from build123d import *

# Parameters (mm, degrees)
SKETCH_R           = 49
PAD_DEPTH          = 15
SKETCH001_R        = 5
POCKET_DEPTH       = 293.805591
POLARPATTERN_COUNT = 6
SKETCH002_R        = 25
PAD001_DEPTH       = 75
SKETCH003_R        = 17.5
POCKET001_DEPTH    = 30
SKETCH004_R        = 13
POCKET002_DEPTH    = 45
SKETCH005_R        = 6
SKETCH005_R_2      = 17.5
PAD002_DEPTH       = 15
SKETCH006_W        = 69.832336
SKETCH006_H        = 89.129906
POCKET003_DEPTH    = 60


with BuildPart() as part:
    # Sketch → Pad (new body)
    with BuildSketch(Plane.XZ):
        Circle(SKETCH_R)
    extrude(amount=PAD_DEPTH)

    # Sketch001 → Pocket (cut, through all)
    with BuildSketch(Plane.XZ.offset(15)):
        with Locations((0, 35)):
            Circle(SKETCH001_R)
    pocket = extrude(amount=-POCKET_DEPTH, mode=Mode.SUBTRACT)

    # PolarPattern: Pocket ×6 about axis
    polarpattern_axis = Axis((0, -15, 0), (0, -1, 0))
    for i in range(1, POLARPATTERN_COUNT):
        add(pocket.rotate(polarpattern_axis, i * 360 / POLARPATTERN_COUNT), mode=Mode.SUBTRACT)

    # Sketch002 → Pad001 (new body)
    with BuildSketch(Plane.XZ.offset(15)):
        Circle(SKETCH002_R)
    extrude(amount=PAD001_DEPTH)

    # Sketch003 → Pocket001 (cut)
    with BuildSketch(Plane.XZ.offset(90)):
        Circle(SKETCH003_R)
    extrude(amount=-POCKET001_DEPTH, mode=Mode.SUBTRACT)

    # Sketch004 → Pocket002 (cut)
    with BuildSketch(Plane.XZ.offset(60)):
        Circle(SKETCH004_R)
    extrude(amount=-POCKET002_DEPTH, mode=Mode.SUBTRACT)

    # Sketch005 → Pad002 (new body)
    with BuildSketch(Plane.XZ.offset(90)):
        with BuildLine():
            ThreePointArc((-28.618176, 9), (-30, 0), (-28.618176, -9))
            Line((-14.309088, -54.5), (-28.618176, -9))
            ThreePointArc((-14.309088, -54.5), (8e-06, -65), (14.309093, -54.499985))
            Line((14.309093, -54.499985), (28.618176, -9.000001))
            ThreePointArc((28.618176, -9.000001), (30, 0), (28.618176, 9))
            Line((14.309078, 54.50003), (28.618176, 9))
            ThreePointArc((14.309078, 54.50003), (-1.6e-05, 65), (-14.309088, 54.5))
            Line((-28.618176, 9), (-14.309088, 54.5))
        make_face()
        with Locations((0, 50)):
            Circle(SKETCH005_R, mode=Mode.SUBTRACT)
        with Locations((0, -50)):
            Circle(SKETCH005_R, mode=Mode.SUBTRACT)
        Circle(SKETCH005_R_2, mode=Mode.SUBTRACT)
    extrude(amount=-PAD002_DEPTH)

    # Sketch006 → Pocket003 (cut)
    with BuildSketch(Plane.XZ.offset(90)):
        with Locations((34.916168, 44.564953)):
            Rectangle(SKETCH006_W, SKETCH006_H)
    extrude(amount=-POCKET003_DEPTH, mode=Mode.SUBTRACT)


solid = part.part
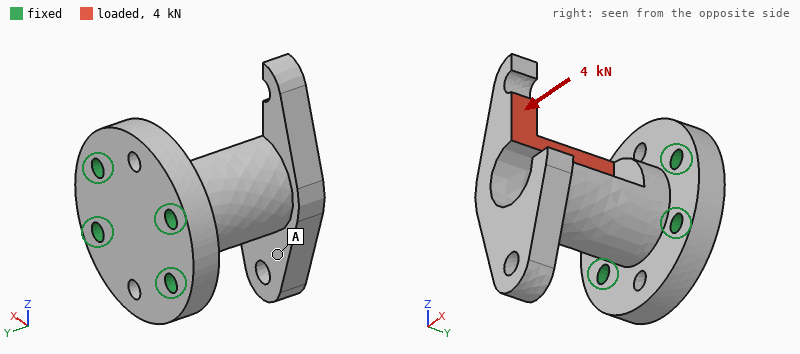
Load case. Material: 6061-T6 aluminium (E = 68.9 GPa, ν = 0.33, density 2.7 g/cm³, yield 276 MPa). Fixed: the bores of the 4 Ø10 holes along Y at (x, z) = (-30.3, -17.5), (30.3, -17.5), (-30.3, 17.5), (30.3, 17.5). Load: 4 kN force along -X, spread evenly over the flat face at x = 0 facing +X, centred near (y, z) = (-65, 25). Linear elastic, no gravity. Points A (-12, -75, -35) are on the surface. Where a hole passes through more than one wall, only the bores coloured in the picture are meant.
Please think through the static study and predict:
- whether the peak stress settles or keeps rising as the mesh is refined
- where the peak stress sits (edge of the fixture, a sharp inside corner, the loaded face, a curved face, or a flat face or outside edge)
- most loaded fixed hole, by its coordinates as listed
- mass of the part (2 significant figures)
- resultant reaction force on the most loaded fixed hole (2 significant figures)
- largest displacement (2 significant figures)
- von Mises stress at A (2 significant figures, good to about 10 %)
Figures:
keeps rising
a sharp inside corner
(30.3, 17.5)
590 g
3.0 kN
0.51 mm
7.9 MPa
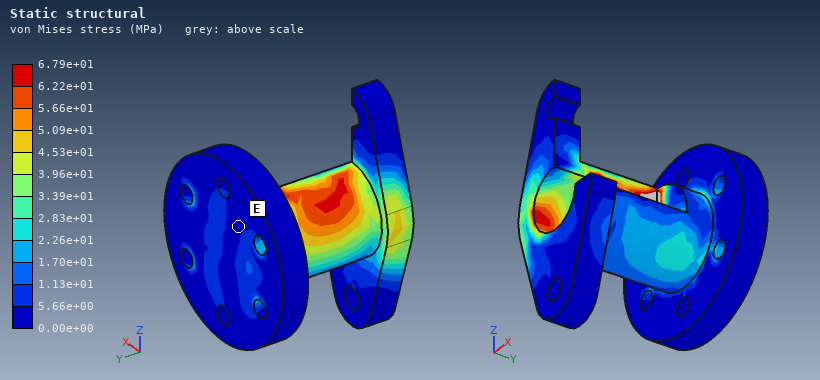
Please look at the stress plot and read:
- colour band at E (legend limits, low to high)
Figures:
0.00e+00 to 5.66e+00 MPa
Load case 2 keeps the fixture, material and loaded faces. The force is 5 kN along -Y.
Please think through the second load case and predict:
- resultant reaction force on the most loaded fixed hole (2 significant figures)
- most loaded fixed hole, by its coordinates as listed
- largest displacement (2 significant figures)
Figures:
3.1 kN
(-30.3, 17.5)
0.14 mm
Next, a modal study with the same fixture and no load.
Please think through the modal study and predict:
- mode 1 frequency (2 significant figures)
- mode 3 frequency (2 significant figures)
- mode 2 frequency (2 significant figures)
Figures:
1800 Hz
3300 Hz
2500 Hz
